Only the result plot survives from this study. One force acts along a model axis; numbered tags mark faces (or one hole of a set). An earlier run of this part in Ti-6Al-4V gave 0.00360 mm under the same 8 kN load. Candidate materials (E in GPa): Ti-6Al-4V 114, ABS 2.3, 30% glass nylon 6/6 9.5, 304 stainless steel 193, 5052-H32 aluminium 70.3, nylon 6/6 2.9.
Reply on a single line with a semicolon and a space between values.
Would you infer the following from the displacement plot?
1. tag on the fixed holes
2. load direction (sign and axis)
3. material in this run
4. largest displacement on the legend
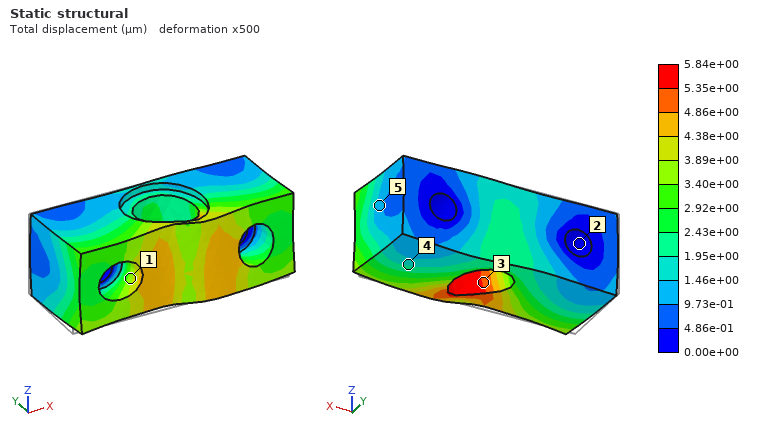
2; +X; 5052-H32 aluminium; 5.84e+00 µm
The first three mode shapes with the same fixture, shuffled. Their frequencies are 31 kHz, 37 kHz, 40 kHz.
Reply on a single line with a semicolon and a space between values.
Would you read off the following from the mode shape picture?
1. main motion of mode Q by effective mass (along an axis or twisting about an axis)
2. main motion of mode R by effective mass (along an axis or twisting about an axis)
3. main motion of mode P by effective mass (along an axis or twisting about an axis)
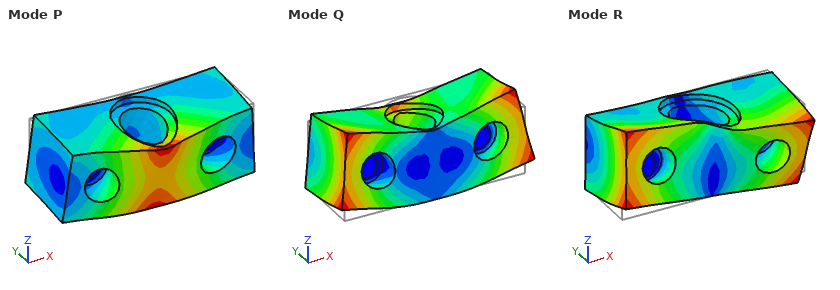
twisting about X; twisting about Y; along Z
